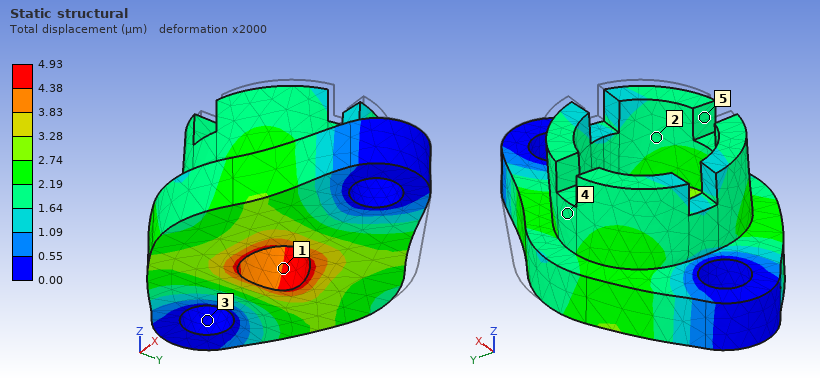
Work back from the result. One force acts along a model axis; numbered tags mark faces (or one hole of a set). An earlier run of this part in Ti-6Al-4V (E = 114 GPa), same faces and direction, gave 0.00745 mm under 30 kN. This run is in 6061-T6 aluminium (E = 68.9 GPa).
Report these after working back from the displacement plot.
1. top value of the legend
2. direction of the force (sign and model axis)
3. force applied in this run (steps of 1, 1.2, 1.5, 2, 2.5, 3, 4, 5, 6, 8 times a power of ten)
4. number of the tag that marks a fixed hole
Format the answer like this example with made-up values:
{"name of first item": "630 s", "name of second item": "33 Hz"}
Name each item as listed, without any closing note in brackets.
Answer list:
{"top value of the legend": "4.93 µm", "direction of the force": "-X", "force applied in this run": "12 kN", "number of the tag that marks a fixed hole": "3"}
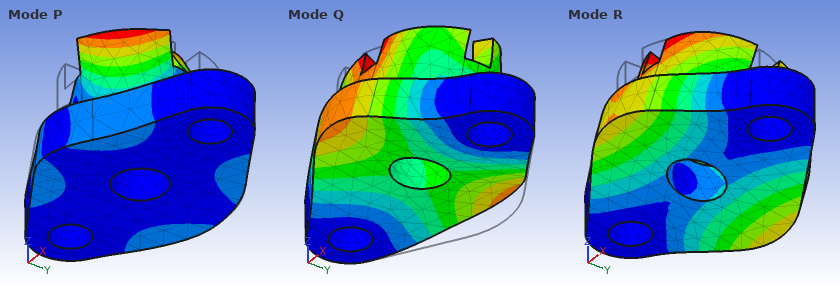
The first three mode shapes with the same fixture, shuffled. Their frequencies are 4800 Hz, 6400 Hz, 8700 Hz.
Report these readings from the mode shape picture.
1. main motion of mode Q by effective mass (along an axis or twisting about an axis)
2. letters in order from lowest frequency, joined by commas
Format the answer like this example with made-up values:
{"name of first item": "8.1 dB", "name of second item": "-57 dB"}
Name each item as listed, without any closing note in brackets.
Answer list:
{"main motion of mode Q by effective mass": "along Z", "letters in order from lowest frequency, joined by commas": "R, Q, P"}
